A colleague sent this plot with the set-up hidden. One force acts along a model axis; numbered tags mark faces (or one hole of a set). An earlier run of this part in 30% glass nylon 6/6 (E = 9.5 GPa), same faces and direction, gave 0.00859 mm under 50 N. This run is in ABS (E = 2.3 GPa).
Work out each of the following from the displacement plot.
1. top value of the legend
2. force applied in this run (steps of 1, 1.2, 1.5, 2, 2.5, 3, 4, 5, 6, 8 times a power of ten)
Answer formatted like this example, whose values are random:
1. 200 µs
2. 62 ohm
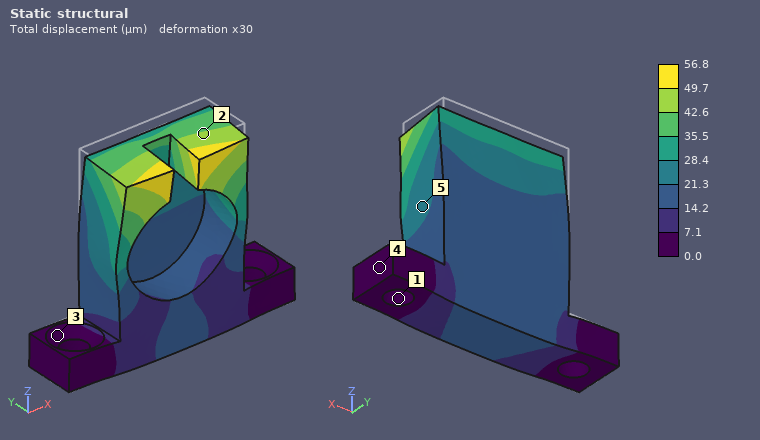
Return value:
1. 56.8 µm
2. 80 N
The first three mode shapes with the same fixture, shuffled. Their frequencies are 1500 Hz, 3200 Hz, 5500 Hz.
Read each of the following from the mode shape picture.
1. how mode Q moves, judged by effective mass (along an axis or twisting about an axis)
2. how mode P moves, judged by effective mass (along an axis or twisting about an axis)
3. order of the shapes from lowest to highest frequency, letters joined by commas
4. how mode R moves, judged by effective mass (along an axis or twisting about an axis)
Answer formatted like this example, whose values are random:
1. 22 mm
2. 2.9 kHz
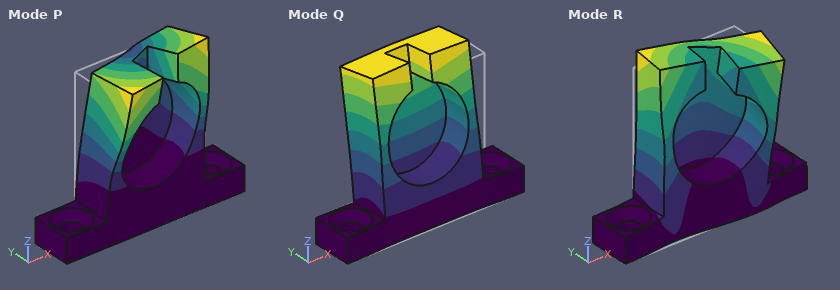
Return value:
1. along Y
2. along X
3. Q, P, R
4. along X
